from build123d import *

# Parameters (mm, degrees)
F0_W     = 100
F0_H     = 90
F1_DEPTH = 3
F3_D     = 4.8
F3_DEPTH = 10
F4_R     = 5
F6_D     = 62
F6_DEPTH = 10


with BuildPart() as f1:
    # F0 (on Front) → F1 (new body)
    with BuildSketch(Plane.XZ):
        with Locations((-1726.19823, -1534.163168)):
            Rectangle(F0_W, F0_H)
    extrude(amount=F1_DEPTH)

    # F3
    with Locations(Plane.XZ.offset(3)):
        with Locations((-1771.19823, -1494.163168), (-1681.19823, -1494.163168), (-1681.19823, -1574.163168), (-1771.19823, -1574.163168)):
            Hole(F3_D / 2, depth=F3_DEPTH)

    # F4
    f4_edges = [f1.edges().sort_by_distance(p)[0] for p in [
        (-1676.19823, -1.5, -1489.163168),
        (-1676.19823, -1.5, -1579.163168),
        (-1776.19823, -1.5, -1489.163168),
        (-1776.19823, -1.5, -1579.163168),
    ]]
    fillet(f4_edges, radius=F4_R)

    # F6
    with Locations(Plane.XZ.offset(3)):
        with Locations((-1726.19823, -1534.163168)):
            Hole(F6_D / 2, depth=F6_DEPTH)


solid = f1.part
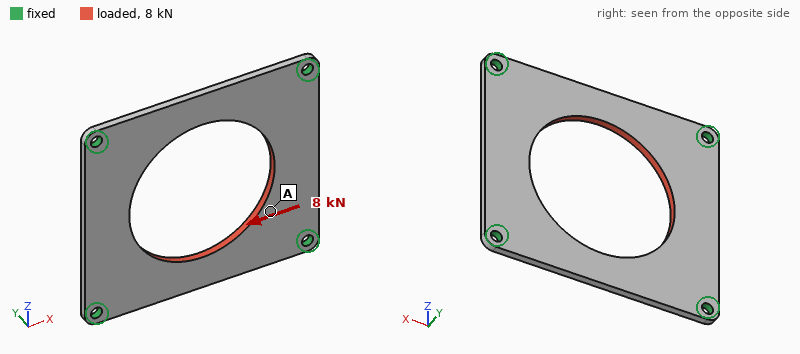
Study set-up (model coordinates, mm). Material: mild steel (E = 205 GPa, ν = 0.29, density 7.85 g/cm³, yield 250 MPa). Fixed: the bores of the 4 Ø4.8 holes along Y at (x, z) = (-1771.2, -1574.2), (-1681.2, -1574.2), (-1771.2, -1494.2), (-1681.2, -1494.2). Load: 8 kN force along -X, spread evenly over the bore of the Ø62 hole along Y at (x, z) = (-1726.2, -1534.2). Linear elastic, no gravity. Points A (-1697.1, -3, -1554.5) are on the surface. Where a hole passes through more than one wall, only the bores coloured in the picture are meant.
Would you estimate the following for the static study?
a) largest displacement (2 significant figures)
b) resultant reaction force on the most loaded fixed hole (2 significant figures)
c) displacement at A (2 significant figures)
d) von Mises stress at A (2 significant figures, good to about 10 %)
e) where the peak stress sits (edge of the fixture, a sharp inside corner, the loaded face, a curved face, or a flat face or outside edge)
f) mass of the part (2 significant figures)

15 µm
2.1 kN
9.6 µm
21 MPa
edge of the fixture
140 g
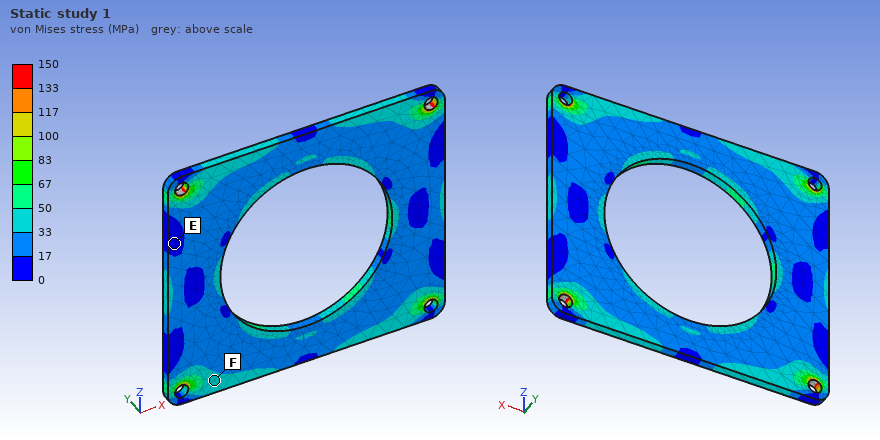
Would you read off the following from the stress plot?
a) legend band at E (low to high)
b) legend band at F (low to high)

0 to 17 MPa
33 to 50 MPa
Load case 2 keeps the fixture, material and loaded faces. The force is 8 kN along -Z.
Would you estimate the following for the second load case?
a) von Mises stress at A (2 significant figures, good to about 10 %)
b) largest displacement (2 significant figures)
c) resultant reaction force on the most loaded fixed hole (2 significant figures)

39 MPa
20 µm
2.1 kN
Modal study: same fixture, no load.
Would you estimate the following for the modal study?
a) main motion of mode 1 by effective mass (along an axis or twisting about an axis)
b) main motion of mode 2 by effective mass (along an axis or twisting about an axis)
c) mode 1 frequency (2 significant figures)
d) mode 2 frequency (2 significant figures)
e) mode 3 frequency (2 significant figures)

along Y
twisting about X
1900 Hz
2200 Hz
2500 Hz
